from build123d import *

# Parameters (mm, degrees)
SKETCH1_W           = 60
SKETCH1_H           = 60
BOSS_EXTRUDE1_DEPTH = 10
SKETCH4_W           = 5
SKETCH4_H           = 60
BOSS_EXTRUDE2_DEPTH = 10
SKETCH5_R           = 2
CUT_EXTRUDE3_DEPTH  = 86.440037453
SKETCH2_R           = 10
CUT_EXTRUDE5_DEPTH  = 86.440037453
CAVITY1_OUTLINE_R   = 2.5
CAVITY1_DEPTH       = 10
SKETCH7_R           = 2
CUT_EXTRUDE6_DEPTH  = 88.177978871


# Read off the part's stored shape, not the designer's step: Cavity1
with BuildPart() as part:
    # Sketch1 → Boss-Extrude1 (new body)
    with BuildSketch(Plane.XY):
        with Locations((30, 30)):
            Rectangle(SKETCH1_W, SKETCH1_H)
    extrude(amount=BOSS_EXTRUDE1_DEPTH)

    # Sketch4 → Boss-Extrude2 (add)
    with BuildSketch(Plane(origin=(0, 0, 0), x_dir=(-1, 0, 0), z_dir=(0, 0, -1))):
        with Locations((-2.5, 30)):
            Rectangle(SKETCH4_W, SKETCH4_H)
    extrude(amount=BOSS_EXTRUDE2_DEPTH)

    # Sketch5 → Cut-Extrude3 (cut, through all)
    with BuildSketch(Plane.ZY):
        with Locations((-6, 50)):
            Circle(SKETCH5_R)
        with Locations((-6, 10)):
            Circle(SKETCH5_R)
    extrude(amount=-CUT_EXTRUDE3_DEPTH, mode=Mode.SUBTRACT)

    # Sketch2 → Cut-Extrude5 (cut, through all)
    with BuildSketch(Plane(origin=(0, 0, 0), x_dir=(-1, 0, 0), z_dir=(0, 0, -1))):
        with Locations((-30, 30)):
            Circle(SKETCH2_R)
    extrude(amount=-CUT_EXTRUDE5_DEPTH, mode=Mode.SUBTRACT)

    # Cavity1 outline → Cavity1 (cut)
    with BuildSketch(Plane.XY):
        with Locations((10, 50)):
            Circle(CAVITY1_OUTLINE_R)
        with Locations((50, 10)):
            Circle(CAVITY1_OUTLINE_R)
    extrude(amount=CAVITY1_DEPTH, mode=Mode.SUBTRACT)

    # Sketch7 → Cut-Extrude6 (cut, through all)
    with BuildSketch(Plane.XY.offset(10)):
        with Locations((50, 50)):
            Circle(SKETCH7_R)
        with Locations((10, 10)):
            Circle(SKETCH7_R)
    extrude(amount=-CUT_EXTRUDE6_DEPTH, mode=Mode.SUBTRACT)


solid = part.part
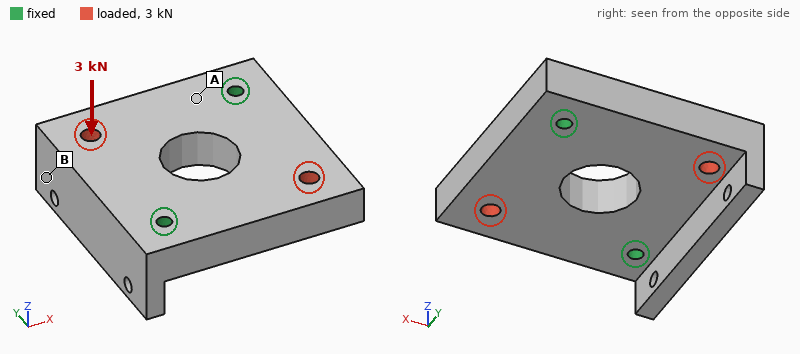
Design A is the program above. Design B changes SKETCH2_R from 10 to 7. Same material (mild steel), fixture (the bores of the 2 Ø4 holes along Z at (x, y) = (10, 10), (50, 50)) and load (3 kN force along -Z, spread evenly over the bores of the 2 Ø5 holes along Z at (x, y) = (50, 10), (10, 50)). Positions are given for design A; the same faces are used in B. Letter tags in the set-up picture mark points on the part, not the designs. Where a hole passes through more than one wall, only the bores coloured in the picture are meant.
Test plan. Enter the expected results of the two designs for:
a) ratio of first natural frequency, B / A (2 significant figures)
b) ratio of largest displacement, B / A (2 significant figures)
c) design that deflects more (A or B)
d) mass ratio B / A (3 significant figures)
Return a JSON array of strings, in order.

["1.0", "0.91", "A", "1.05"]
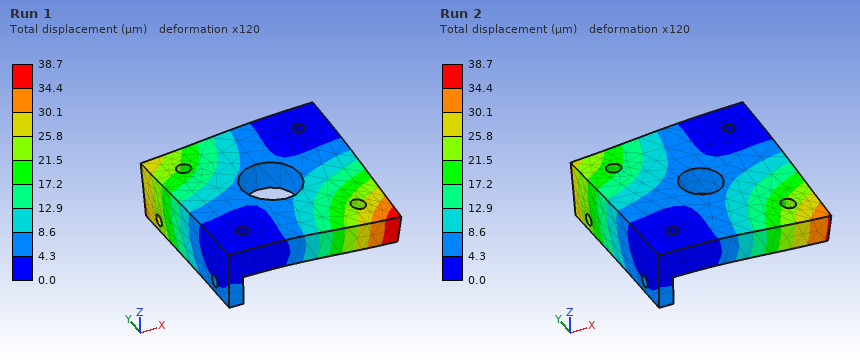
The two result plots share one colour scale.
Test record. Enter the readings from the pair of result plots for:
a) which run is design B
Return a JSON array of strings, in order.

["Run 2"]
